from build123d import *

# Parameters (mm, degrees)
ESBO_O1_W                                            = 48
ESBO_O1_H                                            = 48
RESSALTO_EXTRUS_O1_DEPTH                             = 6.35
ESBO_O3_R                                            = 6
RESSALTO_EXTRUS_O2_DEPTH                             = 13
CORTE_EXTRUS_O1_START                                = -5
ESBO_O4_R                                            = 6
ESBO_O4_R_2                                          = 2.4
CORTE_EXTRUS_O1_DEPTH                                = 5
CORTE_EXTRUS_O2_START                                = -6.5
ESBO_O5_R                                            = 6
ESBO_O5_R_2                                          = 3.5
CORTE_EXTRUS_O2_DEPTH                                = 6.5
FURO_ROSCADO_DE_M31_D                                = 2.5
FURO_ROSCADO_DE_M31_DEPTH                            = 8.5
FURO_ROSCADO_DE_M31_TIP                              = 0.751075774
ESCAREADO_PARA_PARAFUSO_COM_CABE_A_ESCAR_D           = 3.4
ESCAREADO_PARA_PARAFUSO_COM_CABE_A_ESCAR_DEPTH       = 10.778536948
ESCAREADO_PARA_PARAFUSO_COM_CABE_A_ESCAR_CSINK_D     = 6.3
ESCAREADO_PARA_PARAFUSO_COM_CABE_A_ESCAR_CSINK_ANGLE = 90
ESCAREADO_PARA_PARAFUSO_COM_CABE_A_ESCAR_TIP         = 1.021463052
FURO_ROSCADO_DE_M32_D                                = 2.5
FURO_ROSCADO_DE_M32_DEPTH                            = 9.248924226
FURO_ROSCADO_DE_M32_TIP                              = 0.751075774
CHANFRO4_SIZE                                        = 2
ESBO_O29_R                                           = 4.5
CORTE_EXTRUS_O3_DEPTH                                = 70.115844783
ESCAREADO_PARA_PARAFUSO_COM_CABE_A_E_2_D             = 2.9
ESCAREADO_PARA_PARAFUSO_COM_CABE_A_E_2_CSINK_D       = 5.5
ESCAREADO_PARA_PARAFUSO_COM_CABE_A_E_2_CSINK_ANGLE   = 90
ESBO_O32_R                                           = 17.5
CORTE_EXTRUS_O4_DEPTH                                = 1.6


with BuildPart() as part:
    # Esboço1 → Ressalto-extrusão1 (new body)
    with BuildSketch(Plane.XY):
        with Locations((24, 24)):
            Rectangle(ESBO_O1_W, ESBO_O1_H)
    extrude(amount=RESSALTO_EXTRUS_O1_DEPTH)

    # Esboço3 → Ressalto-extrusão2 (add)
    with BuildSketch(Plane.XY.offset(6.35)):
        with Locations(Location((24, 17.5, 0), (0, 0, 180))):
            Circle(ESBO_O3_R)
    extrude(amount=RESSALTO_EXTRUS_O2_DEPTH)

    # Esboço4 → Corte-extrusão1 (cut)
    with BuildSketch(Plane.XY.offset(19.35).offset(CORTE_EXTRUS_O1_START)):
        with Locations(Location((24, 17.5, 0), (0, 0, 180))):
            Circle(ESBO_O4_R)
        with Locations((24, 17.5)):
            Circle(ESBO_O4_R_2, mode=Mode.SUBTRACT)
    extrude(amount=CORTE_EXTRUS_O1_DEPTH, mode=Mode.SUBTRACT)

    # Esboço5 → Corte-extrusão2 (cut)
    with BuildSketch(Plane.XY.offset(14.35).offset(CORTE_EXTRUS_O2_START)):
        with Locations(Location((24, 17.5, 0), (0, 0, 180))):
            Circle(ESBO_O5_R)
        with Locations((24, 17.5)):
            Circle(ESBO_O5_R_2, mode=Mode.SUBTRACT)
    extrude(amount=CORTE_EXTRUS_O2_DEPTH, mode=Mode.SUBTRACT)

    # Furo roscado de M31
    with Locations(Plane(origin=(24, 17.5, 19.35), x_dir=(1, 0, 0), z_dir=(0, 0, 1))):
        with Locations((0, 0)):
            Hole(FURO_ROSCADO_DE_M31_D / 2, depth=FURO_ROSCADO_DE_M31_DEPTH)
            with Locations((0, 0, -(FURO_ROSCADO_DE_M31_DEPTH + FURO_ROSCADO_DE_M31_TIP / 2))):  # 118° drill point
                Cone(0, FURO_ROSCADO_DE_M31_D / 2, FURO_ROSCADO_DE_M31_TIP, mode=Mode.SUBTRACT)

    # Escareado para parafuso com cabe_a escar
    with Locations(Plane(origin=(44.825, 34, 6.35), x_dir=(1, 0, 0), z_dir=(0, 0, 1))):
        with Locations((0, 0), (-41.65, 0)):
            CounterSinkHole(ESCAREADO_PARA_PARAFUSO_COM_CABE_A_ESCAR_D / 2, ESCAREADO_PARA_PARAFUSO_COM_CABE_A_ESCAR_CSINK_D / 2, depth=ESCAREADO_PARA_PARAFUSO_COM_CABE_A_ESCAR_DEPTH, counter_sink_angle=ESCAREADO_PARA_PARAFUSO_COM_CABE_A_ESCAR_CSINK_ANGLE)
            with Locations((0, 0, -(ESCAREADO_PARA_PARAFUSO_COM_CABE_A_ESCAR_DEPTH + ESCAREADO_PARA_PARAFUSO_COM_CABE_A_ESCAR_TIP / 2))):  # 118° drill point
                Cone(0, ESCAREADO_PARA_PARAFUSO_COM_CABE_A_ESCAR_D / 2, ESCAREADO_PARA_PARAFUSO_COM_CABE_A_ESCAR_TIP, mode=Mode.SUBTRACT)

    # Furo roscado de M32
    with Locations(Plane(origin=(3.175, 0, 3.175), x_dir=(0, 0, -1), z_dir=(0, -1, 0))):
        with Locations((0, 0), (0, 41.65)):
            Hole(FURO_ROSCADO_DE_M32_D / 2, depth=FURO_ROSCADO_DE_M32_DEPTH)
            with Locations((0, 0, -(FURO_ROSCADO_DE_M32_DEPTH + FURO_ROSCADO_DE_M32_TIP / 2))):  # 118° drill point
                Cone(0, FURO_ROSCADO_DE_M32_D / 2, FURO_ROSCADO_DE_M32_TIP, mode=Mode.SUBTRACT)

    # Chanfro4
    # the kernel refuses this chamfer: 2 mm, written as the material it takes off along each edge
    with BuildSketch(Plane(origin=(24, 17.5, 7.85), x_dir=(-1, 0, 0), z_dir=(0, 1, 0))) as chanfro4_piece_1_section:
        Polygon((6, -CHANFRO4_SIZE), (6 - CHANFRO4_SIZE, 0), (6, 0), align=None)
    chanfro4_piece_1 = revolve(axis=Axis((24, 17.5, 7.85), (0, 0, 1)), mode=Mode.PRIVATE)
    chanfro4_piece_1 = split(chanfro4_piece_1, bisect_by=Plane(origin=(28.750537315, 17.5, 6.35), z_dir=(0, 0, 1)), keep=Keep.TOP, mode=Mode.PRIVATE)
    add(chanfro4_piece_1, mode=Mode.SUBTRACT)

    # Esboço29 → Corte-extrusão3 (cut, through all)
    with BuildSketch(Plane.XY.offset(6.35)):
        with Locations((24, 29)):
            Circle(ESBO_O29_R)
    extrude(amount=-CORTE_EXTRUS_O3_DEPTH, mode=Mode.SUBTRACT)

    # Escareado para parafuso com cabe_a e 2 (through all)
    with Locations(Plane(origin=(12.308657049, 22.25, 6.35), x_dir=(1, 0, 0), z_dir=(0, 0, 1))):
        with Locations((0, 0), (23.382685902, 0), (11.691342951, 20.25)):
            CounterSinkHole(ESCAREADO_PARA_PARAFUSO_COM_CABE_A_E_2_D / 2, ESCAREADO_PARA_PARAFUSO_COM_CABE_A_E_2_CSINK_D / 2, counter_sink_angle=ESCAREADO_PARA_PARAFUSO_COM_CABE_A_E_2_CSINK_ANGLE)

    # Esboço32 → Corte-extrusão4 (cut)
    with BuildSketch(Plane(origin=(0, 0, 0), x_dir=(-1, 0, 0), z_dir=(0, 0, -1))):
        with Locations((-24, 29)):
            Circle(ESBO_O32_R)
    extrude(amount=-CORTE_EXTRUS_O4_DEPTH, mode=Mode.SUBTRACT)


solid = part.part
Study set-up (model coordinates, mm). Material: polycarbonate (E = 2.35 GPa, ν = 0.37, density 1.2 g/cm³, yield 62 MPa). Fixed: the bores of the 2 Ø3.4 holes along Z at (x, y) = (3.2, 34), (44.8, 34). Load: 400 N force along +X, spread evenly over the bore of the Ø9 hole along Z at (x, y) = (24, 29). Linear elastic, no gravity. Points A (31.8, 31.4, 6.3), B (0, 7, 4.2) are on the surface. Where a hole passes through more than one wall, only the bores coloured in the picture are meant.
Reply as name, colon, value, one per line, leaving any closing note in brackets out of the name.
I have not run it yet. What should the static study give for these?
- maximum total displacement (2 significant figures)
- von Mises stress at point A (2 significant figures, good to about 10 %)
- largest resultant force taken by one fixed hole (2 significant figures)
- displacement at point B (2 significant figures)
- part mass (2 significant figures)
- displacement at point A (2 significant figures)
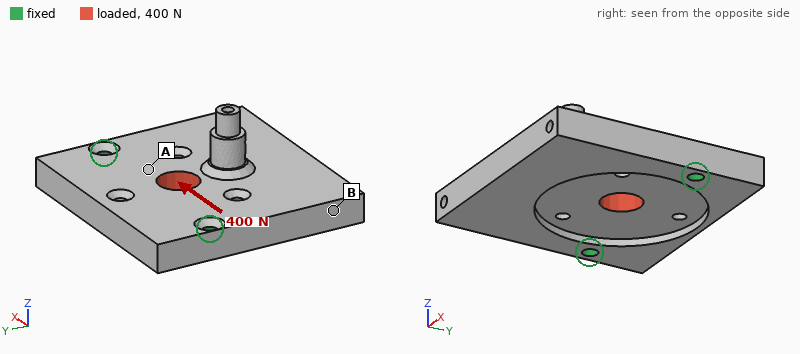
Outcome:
maximum total displacement: 36 µm
von Mises stress at point A: 3.1 MPa
largest resultant force taken by one fixed hole: 210 N
displacement at point B: 26 µm
part mass: 15 g
displacement at point A: 21 µm
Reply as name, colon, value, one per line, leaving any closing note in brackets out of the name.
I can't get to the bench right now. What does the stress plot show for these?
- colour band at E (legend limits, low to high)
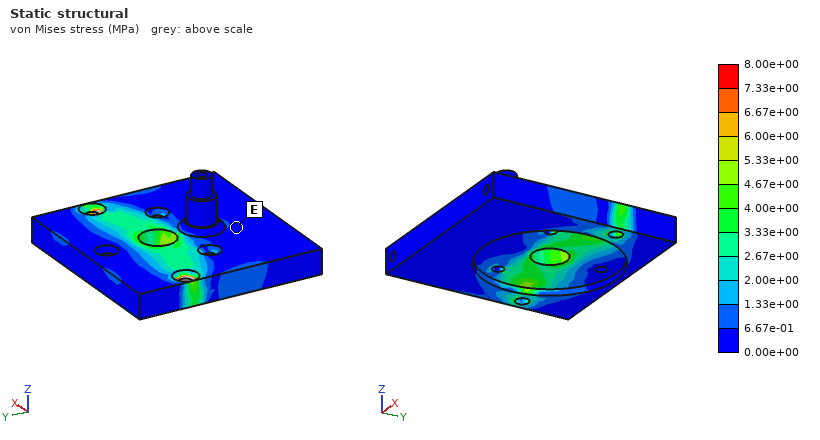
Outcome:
colour band at E: 0.00e+00 to 6.67e-01 MPa
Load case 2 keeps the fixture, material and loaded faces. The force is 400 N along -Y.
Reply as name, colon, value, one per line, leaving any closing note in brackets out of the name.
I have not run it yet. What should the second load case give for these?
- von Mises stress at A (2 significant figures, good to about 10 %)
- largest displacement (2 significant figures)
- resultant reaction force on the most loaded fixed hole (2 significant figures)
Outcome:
von Mises stress at A: 2.1 MPa
largest displacement: 0.10 mm
resultant reaction force on the most loaded fixed hole: 200 N
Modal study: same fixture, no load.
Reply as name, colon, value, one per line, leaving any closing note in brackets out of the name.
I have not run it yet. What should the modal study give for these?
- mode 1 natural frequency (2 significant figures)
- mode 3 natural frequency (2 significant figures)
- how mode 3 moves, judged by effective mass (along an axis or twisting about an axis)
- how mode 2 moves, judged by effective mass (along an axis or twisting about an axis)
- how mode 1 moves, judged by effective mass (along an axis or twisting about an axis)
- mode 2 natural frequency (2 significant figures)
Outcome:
mode 1 natural frequency: 780 Hz
mode 3 natural frequency: 3000 Hz
how mode 3 moves, judged by effective mass: along Z
how mode 2 moves, judged by effective mass: twisting about Y
how mode 1 moves, judged by effective mass: along Z
mode 2 natural frequency: 1900 Hz
